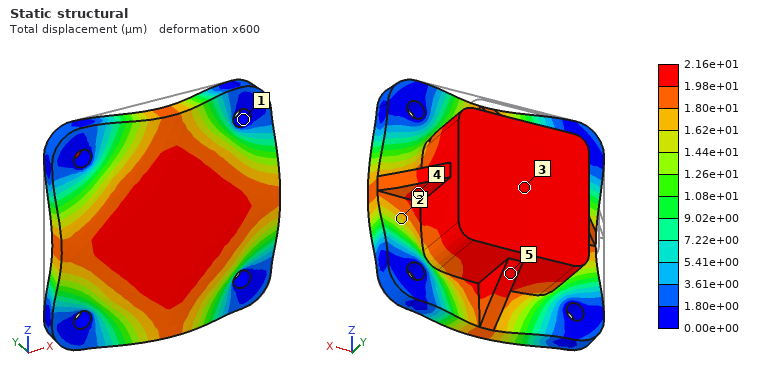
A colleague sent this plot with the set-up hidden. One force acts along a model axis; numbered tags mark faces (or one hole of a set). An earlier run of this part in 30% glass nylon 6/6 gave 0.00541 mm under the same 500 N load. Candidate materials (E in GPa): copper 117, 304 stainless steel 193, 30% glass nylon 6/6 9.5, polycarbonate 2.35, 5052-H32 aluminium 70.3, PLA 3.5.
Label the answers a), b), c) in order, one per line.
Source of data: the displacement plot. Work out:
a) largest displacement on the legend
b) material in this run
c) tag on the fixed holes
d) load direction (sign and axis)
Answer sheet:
a) 2.16e+01 µm
b) polycarbonate
c) 1
d) -Y
